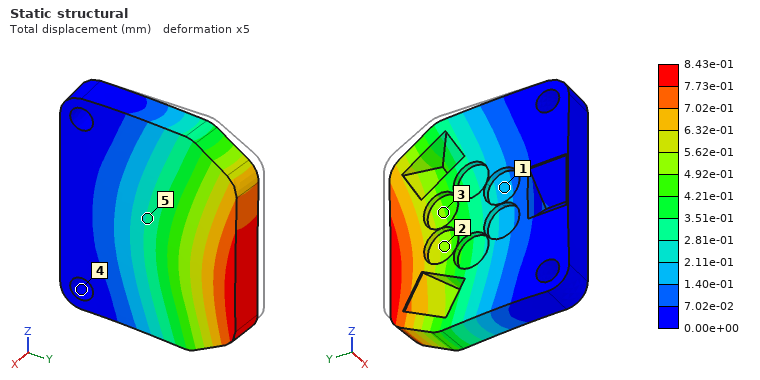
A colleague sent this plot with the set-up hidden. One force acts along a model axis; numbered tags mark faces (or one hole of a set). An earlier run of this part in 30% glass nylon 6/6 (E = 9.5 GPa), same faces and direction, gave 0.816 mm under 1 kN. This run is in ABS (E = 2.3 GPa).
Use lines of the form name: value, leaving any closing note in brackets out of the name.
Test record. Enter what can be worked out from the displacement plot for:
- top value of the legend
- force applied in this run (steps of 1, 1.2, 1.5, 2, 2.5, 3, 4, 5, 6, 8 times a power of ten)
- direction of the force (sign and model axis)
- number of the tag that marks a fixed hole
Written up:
top value of the legend: 8.43e-01 mm
force applied in this run: 250 N
direction of the force: +X
number of the tag that marks a fixed hole: 4
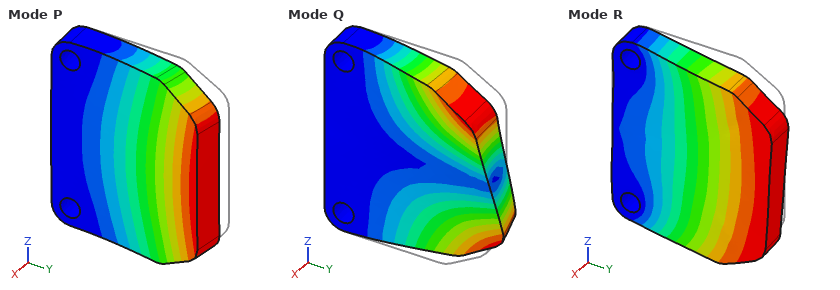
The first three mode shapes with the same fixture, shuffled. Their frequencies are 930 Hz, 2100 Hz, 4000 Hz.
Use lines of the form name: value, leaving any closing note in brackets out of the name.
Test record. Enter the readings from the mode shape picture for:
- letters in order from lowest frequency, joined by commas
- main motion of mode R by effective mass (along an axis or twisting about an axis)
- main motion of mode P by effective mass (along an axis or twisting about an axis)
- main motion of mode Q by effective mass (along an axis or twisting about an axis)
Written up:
letters in order from lowest frequency, joined by commas: P, Q, R
main motion of mode R by effective mass: along Z
main motion of mode P by effective mass: along X
main motion of mode Q by effective mass: twisting about Y
